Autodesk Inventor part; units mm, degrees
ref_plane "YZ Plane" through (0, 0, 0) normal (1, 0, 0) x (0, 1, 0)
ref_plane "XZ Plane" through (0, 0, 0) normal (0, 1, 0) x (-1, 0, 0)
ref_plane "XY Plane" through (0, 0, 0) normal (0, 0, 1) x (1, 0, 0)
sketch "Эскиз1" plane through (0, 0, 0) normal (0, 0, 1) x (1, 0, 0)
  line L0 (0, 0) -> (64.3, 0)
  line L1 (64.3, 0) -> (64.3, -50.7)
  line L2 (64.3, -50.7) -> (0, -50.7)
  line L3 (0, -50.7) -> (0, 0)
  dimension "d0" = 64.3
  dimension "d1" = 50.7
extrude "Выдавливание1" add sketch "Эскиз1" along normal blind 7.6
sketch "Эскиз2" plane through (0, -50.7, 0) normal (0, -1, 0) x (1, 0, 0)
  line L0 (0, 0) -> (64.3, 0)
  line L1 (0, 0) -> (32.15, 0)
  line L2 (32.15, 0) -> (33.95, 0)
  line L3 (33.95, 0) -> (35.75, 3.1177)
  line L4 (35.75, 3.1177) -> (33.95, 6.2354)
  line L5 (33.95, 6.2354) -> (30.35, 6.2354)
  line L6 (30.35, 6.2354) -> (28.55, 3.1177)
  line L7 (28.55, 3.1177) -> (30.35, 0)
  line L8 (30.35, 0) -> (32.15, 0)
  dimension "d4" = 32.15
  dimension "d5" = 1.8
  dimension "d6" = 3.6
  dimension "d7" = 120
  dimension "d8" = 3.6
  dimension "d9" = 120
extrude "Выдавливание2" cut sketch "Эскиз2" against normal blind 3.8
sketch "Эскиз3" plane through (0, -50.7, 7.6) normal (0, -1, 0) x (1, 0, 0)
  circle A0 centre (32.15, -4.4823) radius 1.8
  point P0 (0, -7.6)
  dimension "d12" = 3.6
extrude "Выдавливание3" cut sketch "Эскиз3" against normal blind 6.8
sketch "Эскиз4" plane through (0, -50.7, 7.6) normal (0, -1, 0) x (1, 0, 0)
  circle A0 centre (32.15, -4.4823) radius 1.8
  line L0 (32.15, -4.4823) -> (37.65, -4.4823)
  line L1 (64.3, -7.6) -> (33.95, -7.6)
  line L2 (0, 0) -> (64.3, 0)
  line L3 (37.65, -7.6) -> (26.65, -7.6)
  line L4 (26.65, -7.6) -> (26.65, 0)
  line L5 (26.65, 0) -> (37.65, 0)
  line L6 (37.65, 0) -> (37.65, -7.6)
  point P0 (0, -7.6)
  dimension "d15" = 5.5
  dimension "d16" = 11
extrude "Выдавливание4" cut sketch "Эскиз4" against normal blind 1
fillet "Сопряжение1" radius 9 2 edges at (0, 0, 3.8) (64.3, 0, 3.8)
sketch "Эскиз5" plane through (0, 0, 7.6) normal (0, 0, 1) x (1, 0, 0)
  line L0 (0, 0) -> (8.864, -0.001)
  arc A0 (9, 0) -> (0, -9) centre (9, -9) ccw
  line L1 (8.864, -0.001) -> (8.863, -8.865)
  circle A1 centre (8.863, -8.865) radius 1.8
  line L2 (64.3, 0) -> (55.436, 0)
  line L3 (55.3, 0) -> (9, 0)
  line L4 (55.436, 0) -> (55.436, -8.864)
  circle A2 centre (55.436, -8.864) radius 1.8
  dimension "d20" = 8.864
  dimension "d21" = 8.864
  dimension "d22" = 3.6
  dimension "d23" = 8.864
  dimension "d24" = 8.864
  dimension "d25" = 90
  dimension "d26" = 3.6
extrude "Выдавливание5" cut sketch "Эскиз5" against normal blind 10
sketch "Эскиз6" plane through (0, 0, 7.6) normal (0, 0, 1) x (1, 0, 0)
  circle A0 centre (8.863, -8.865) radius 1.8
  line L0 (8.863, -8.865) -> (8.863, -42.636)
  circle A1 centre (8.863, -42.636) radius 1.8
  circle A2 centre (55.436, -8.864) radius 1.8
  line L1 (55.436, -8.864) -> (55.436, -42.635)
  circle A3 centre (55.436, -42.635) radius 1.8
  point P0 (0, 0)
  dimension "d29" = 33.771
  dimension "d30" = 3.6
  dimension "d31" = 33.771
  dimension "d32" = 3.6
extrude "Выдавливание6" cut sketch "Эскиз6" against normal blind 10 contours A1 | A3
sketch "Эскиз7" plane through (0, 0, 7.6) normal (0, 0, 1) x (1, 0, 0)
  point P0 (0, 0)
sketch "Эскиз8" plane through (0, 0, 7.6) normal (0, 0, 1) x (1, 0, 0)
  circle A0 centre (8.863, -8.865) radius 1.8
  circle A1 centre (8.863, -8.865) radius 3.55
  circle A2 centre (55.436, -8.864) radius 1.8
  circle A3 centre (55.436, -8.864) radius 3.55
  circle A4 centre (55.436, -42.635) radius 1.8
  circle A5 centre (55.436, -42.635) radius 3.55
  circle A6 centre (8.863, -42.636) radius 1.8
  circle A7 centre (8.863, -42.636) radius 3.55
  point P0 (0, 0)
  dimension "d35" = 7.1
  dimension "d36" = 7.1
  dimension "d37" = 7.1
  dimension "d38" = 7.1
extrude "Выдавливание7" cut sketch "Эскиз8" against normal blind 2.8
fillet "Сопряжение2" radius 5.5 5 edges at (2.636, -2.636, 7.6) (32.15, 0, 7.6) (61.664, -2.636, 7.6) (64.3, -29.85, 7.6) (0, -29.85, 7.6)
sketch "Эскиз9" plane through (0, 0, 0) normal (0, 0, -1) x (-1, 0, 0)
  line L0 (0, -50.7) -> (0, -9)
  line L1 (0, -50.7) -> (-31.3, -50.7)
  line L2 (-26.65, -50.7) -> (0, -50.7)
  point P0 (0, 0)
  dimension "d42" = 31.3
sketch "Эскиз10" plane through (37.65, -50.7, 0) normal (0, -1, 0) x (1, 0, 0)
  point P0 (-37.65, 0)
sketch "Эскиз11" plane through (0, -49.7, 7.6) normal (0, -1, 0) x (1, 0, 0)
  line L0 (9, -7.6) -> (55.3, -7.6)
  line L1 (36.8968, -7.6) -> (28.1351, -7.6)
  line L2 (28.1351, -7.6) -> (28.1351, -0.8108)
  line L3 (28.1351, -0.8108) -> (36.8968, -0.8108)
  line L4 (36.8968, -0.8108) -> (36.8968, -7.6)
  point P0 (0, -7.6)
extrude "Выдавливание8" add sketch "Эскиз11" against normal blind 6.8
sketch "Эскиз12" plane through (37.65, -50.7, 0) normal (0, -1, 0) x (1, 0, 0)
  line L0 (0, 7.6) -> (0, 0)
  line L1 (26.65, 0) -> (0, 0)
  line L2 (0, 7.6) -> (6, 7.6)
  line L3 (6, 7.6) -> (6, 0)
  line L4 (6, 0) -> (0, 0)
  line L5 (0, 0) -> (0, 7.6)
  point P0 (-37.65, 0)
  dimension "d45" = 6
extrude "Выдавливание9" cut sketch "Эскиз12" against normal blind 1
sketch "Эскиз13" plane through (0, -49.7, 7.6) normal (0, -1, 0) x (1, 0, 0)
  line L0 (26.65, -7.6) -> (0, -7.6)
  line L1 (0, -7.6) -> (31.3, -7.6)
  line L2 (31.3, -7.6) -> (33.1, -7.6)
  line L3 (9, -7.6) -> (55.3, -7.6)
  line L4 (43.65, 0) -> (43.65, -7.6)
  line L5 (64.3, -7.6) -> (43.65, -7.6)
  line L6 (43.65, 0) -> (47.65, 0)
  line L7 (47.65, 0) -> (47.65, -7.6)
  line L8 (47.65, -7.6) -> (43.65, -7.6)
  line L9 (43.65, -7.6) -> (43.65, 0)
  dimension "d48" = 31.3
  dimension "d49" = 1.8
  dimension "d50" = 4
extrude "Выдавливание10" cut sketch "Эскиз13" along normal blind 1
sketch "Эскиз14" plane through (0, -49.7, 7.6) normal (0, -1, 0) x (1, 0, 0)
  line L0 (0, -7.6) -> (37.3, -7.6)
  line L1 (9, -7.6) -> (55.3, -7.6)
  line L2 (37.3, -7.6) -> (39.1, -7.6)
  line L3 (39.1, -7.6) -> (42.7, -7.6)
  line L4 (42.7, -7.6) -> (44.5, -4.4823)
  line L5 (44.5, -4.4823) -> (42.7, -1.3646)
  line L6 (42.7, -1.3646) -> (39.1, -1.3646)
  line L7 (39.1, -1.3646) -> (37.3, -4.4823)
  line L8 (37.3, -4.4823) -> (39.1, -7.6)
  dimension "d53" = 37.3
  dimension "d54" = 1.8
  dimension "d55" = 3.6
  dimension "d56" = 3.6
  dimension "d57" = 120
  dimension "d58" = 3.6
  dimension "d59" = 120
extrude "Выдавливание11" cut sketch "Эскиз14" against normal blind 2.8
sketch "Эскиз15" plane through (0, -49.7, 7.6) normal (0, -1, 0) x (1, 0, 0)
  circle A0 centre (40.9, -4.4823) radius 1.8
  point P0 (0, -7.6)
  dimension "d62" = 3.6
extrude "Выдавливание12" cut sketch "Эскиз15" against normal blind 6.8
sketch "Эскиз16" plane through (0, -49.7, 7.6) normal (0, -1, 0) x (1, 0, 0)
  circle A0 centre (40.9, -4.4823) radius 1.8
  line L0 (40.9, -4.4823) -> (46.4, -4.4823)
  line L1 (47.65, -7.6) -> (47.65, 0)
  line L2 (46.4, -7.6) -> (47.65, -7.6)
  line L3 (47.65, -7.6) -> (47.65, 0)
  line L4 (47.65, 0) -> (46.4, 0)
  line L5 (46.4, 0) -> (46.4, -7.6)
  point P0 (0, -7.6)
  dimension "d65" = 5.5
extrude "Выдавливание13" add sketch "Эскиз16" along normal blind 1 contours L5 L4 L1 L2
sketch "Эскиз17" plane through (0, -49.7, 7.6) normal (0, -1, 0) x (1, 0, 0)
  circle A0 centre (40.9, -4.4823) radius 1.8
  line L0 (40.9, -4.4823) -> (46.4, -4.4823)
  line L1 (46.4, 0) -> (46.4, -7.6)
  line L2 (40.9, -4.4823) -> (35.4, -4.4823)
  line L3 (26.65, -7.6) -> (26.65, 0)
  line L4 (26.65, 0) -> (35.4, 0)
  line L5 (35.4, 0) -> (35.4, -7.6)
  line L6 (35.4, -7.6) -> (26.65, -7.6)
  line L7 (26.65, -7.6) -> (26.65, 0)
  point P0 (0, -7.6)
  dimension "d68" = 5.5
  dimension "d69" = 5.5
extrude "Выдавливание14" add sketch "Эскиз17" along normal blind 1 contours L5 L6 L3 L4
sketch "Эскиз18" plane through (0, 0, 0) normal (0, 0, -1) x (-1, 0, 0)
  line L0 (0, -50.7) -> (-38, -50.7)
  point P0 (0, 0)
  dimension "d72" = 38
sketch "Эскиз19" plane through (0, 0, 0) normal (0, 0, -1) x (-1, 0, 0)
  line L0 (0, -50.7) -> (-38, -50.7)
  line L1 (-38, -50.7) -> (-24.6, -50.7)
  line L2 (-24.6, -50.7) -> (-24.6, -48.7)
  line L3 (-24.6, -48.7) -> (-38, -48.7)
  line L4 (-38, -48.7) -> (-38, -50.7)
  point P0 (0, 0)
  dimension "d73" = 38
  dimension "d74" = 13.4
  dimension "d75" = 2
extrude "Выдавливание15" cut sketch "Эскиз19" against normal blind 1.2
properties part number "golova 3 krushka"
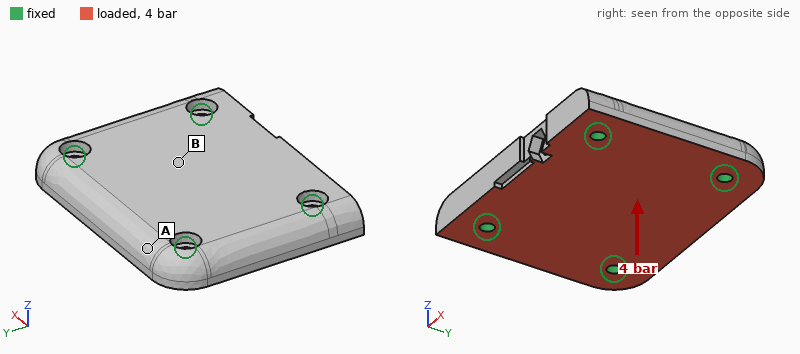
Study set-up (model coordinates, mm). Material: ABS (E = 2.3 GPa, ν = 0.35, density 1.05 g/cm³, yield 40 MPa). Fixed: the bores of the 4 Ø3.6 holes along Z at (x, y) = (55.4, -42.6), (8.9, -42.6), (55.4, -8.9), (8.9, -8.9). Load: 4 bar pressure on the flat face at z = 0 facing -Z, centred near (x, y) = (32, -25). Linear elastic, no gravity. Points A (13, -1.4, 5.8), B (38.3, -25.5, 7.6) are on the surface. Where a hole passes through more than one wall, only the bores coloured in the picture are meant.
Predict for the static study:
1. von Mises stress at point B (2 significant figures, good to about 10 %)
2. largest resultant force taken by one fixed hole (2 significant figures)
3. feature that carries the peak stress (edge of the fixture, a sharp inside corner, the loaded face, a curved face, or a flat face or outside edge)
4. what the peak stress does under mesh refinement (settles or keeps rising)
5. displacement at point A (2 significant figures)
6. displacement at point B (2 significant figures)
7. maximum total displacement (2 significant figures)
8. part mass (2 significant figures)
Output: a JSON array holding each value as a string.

["4.5 MPa", "340 N", "edge of the fixture", "keeps rising", "0.040 mm", "0.14 mm", "0.15 mm", "24 g"]
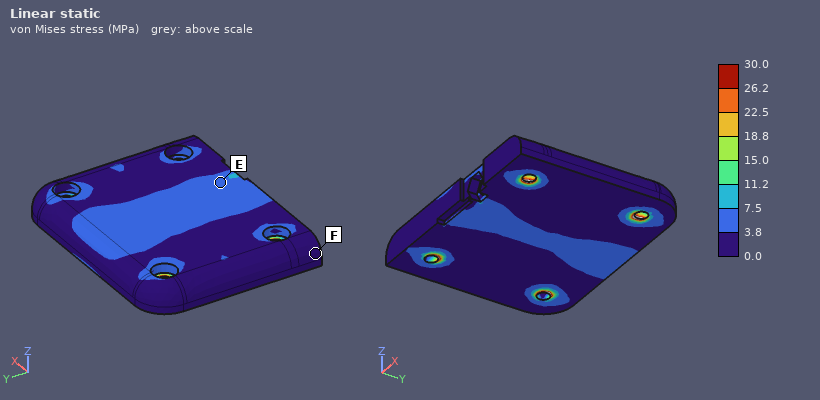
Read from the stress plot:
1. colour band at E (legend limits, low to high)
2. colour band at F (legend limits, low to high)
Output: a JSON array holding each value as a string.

["3.8 to 7.5 MPa", "0.0 to 3.8 MPa"]
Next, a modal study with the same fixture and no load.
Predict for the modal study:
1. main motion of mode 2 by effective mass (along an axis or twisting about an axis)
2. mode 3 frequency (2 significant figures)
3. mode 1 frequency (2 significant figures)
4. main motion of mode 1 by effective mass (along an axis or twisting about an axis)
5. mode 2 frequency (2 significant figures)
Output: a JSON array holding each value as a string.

["twisting about X", "5600 Hz", "3200 Hz", "along Z", "4300 Hz"]
